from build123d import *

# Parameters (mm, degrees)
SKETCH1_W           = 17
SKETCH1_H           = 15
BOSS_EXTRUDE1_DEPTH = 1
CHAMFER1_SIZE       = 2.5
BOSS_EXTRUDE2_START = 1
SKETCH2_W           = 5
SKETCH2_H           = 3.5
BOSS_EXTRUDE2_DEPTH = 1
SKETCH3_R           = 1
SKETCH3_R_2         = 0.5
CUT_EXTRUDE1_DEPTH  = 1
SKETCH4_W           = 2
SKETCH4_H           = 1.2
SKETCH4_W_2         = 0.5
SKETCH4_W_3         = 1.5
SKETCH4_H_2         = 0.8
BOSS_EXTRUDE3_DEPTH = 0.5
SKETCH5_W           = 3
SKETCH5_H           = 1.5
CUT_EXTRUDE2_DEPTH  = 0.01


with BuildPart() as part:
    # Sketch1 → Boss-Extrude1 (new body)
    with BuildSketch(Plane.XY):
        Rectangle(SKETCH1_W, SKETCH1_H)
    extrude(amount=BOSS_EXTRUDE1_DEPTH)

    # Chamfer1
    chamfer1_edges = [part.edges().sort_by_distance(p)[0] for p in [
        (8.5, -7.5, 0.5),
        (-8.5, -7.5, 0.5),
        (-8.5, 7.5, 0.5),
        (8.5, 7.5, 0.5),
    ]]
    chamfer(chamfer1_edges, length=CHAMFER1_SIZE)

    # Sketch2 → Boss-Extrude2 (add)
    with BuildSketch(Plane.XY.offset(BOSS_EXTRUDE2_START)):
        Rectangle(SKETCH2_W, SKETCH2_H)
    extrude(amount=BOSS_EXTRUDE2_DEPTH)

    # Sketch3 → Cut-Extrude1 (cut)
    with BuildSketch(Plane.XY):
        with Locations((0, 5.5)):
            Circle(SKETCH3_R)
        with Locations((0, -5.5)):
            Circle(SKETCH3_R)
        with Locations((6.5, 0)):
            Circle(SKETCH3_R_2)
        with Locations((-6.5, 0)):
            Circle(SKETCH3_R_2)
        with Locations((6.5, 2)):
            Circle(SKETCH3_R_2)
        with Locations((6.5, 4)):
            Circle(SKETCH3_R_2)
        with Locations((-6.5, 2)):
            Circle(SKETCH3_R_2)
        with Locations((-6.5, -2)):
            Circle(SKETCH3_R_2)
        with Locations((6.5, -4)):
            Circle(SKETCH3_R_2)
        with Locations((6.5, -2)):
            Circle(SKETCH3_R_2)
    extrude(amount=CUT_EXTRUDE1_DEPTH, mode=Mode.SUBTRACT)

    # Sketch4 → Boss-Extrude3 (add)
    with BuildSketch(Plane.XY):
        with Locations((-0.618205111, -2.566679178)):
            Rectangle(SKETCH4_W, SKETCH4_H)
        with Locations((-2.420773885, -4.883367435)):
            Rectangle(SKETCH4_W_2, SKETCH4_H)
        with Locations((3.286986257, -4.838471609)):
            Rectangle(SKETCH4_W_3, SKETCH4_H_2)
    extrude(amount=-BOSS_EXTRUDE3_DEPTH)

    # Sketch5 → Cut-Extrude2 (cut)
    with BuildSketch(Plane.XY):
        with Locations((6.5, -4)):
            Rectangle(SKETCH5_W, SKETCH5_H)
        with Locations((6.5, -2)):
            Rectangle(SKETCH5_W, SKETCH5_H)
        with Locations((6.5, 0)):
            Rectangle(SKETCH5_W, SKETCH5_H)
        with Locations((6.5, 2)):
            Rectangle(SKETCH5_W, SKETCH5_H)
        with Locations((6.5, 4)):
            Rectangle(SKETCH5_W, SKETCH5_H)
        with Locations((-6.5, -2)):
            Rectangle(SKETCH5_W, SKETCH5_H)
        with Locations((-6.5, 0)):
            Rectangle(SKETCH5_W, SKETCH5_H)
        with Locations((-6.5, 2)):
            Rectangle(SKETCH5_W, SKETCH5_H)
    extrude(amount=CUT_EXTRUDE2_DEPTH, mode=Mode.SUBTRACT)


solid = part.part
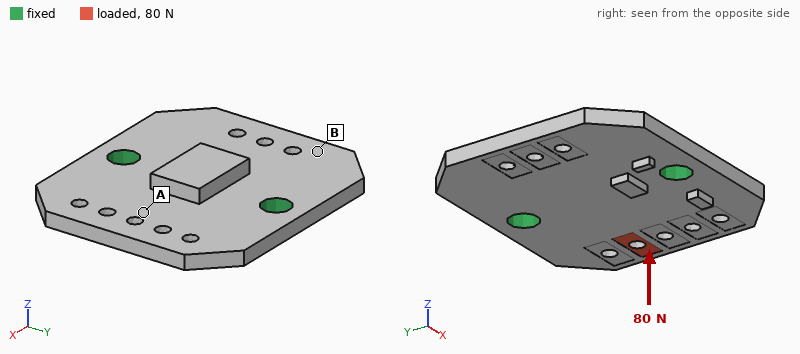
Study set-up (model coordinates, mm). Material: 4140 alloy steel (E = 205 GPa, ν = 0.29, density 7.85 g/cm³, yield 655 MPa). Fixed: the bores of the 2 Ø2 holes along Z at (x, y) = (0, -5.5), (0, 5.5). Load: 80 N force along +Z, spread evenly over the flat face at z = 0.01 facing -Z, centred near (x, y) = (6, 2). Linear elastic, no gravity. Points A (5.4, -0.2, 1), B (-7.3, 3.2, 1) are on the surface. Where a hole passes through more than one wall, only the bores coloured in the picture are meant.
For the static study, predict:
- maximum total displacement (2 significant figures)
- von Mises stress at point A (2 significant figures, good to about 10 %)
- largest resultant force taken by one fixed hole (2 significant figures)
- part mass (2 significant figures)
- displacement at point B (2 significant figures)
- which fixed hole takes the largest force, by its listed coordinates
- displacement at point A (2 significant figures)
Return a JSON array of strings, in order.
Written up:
["45 µm", "78 MPa", "61 N", "2.0 g", "7.6 µm", "(0, 5.5)", "21 µm"]
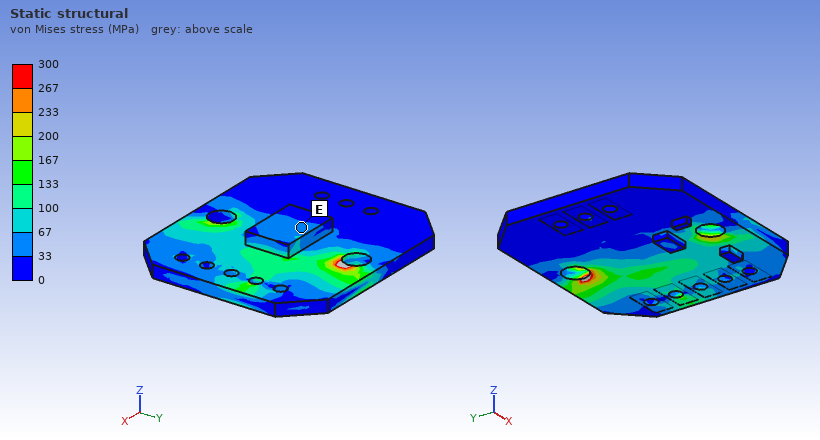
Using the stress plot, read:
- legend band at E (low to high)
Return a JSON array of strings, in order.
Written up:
["33 to 67 MPa"]
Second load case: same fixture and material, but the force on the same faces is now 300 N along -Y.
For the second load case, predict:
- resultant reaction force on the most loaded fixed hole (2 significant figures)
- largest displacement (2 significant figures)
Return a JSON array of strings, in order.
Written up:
["220 N", "9.3 µm"]
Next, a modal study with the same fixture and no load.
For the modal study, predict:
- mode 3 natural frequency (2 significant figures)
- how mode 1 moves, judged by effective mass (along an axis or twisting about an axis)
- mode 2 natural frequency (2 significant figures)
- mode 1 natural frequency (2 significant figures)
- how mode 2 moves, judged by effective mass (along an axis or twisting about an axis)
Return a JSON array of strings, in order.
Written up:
["25 kHz", "twisting about Y", "16 kHz", "12 kHz", "along Z"]
